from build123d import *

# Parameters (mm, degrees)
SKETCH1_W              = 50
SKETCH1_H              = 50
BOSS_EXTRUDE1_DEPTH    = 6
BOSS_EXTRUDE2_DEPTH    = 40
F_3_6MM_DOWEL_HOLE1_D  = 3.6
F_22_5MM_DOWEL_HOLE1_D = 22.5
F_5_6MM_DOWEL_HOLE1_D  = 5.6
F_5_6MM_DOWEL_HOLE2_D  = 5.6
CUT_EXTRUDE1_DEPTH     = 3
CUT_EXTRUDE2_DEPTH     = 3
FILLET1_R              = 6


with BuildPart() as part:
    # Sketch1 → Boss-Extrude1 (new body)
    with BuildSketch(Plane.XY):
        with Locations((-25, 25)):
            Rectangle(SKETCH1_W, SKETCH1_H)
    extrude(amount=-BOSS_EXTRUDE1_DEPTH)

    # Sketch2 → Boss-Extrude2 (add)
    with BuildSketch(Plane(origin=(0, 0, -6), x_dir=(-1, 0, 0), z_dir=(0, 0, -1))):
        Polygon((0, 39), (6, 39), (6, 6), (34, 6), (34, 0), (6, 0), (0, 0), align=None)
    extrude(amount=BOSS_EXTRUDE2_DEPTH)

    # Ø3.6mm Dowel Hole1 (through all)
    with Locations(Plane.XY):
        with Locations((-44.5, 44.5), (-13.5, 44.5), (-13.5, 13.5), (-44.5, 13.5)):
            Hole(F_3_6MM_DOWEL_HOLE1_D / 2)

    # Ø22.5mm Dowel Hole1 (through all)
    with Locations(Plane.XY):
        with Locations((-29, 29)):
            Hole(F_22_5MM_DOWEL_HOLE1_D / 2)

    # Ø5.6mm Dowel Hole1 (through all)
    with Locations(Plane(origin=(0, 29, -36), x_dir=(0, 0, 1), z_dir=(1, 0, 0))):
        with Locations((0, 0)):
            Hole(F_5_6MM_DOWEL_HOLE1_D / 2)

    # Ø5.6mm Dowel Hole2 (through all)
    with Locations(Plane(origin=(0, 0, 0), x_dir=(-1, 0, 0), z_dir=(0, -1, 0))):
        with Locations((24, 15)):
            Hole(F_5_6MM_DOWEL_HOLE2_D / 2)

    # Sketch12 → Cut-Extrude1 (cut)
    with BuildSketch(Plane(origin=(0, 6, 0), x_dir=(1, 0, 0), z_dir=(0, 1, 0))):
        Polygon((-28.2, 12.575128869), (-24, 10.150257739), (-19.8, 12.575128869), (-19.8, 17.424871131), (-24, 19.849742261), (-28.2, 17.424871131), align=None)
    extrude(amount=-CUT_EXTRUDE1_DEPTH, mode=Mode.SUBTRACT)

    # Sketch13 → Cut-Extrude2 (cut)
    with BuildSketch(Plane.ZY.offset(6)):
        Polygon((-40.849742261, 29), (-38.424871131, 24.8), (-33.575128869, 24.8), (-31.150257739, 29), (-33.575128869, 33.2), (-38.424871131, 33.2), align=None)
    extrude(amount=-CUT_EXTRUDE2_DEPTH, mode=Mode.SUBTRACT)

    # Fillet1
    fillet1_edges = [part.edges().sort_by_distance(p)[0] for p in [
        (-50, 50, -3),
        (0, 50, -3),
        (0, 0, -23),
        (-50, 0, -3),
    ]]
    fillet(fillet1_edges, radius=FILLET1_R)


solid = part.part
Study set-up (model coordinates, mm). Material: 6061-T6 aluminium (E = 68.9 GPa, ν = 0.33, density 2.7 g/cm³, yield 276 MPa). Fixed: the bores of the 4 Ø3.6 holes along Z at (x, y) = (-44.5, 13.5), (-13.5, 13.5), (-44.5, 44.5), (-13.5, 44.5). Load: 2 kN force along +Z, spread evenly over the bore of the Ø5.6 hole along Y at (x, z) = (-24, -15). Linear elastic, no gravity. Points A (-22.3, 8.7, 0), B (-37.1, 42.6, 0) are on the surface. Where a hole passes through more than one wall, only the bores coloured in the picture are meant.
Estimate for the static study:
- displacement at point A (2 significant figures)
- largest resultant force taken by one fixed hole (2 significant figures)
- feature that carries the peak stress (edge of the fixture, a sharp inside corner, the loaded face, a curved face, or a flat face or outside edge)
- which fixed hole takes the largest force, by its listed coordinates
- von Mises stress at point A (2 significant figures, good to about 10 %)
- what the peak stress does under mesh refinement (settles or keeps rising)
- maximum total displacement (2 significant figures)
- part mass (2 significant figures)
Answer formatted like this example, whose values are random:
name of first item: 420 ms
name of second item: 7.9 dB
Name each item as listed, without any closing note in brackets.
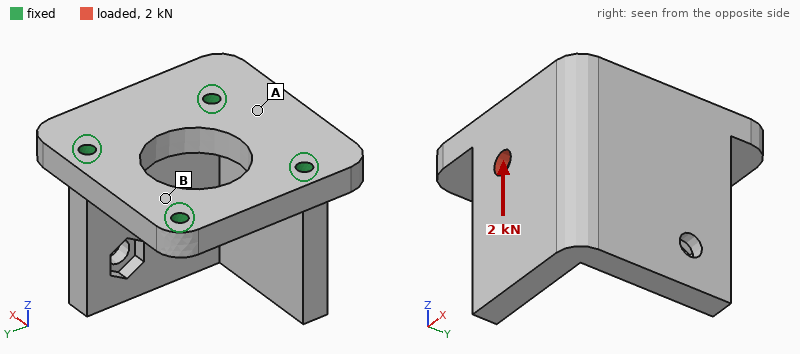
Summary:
displacement at point A: 15 µm
largest resultant force taken by one fixed hole: 1.7 kN
feature that carries the peak stress: edge of the fixture
which fixed hole takes the largest force, by its listed coordinates: (-13.5, 13.5)
von Mises stress at point A: 22 MPa
what the peak stress does under mesh refinement: keeps rising
maximum total displacement: 80 µm
part mass: 74 g
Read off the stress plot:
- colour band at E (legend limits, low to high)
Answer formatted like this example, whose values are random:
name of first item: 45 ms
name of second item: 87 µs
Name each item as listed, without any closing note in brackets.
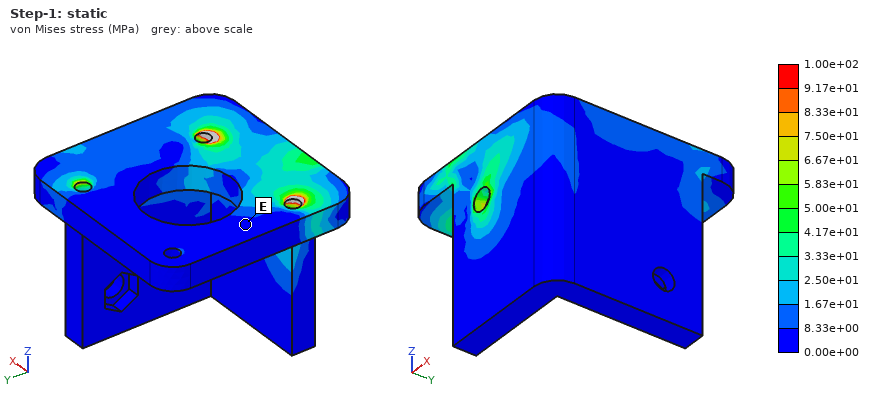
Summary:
colour band at E: 0.00e+00 to 8.33e+00 MPa
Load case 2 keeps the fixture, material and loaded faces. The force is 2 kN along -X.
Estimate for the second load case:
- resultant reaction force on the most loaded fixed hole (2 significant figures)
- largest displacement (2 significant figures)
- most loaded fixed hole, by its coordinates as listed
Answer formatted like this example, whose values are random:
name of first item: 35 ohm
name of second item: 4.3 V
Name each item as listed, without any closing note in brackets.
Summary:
resultant reaction force on the most loaded fixed hole: 1.5 kN
largest displacement: 65 µm
most loaded fixed hole, by its coordinates as listed: (-13.5, 13.5)
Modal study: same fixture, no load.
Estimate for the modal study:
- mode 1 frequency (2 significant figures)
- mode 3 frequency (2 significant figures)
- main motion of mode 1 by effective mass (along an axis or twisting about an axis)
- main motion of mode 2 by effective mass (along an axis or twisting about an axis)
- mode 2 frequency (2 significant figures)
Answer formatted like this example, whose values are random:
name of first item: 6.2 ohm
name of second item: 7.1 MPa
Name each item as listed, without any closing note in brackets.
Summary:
mode 1 frequency: 3200 Hz
mode 3 frequency: 7000 Hz
main motion of mode 1 by effective mass: along X
main motion of mode 2 by effective mass: along Y
mode 2 frequency: 3600 Hz
